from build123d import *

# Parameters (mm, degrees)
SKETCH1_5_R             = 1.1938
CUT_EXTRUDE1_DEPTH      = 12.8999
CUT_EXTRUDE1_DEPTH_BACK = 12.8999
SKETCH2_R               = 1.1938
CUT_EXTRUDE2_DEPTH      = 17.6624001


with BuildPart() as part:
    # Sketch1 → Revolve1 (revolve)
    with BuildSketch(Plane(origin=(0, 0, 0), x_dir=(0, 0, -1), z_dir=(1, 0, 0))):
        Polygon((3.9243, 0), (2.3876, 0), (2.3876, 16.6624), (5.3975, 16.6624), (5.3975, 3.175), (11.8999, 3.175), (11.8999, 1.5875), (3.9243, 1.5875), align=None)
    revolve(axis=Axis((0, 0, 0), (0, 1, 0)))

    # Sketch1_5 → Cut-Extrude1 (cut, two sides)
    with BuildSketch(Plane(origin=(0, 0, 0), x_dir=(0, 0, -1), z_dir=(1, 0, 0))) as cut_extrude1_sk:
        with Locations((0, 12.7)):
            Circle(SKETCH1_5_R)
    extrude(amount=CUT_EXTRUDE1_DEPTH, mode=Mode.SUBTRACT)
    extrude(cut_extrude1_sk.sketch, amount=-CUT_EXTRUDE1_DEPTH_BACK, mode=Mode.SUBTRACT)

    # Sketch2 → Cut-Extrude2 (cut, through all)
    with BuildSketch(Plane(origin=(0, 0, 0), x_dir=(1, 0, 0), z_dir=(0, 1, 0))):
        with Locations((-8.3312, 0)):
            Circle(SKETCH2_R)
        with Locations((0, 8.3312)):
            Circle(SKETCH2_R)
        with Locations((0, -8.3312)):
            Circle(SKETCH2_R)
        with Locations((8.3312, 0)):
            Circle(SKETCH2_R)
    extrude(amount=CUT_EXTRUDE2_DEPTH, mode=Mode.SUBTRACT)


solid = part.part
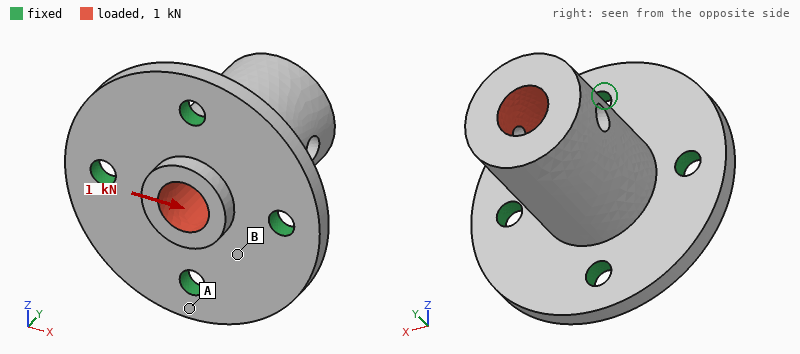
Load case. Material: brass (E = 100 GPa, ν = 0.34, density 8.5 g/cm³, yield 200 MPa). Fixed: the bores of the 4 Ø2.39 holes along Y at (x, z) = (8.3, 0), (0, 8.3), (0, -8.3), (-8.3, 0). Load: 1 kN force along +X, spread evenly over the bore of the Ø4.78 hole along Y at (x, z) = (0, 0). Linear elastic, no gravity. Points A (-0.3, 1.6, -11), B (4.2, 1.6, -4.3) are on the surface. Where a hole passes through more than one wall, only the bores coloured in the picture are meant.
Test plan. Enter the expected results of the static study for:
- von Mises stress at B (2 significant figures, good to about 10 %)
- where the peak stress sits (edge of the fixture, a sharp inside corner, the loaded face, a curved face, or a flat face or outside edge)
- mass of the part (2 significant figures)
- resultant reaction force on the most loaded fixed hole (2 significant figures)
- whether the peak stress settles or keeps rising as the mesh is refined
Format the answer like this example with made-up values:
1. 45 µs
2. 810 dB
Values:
1. 44 MPa
2. edge of the fixture
3. 14 g
4. 530 N
5. keeps rising
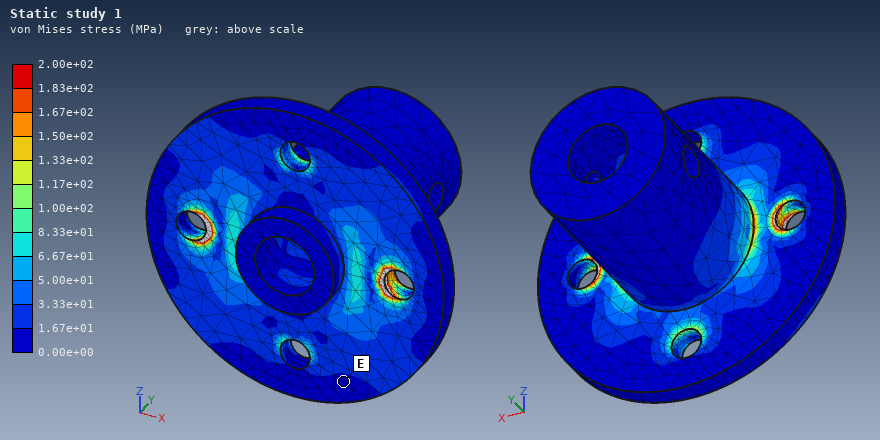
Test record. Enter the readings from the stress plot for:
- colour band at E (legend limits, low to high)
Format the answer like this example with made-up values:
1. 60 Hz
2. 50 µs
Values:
1. 0.00e+00 to 1.67e+01 MPa
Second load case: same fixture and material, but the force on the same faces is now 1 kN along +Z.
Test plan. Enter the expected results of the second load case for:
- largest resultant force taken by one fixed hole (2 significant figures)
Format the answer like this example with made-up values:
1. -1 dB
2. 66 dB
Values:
1. 530 N
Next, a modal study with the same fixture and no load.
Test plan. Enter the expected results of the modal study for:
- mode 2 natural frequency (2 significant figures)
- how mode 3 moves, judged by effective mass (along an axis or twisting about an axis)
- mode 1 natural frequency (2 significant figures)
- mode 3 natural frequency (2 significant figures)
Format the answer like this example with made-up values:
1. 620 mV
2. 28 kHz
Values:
1. 11 kHz
2. along Y
3. 11 kHz
4. 21 kHz
